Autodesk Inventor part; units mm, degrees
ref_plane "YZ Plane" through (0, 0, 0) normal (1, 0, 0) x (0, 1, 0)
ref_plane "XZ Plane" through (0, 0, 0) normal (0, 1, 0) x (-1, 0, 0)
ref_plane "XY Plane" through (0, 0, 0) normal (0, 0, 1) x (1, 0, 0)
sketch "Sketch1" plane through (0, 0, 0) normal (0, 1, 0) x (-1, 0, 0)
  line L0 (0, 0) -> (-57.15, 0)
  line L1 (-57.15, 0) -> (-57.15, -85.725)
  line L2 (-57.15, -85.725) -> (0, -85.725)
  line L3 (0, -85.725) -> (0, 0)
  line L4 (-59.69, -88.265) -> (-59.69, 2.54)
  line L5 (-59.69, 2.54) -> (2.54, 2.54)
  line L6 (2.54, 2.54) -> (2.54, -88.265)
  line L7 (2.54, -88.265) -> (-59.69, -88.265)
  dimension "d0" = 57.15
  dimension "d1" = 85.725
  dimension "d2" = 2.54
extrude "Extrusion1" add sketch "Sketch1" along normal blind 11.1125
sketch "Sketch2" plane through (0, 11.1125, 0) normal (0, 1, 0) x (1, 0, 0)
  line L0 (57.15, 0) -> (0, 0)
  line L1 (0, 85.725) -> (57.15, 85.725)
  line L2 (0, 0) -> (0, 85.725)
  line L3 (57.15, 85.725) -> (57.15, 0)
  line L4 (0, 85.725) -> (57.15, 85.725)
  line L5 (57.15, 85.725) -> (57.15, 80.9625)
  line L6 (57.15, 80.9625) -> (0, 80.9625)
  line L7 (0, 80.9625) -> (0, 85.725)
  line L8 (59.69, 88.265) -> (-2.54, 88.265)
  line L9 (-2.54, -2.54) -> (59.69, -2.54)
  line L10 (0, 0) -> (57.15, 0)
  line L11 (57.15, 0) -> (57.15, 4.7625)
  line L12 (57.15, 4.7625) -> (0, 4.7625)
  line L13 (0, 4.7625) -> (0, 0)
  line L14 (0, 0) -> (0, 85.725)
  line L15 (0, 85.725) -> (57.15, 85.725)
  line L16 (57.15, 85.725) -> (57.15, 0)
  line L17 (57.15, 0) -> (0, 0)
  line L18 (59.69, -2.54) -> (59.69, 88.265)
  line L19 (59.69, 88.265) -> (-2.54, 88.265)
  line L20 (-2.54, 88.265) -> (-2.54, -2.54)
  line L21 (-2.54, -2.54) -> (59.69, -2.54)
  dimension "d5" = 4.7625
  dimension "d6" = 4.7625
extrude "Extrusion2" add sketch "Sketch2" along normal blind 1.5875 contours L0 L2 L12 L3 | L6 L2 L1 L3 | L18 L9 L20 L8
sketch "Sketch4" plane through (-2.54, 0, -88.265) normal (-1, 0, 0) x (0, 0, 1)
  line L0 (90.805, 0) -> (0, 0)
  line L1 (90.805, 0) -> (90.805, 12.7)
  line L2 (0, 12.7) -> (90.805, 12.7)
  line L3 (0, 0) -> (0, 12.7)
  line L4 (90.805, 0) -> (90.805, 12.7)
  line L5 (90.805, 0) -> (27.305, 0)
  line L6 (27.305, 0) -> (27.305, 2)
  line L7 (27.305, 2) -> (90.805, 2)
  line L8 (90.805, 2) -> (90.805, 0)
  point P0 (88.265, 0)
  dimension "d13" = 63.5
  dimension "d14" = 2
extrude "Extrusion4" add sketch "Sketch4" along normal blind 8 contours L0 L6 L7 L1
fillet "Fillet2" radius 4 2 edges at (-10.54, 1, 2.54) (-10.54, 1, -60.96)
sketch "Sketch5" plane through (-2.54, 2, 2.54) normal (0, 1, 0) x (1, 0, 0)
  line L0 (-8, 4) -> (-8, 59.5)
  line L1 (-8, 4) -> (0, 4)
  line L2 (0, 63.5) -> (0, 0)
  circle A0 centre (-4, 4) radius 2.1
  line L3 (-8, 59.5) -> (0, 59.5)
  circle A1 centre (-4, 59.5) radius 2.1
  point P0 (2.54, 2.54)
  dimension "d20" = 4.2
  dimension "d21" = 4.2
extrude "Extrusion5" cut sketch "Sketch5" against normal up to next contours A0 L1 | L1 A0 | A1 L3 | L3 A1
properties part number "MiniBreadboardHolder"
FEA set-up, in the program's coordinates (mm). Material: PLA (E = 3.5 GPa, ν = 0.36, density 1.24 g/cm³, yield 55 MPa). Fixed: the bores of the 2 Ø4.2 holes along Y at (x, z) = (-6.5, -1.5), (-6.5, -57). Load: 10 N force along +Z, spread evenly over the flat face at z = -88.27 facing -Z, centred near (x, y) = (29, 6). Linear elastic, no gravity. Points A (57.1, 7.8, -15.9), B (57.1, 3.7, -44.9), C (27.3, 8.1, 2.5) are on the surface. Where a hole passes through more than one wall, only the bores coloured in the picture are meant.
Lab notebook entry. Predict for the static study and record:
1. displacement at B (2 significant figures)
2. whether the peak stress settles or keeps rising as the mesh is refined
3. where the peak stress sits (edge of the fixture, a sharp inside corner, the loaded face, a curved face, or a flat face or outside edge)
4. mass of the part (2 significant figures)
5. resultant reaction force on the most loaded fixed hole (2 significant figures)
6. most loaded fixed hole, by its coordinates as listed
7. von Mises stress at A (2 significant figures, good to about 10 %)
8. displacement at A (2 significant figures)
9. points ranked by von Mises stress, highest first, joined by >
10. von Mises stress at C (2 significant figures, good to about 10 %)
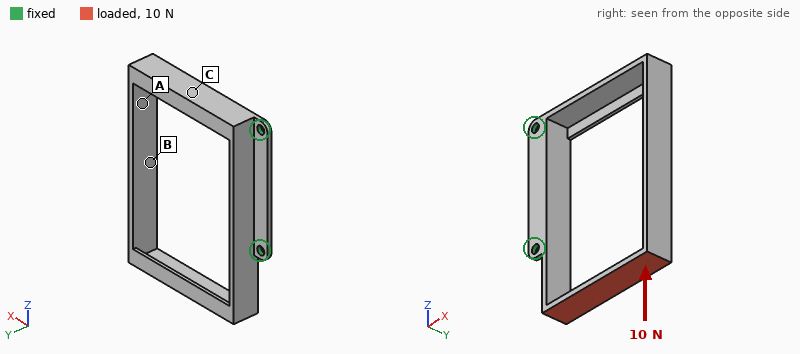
1.2 mm
keeps rising
a sharp inside corner
14 g
7.9 N
(-6.5, -57)
3.0 MPa
1.2 mm
A > C > B
1.6 MPa
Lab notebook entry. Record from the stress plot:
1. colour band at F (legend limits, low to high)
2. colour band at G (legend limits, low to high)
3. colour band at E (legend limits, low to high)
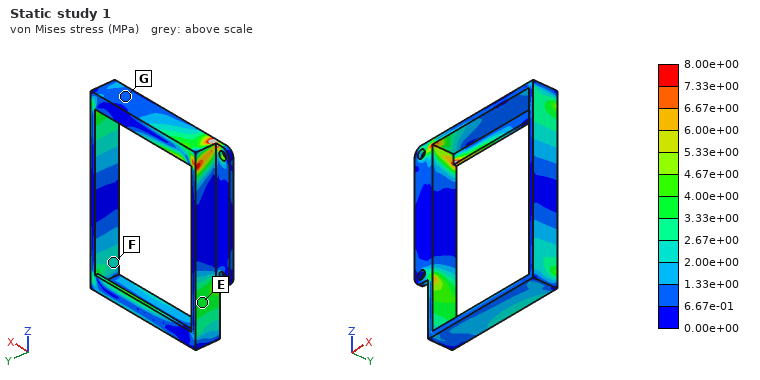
2.00e+00 to 2.67e+00 MPa
6.67e-01 to 1.33e+00 MPa
3.33e+00 to 4.00e+00 MPa
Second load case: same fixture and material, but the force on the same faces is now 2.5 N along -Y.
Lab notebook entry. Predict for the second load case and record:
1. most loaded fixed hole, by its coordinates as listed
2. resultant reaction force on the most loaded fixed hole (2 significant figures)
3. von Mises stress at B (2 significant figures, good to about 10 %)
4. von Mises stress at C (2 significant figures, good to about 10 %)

(-6.5, -57)
4.7 N
0.94 MPa
0.99 MPa
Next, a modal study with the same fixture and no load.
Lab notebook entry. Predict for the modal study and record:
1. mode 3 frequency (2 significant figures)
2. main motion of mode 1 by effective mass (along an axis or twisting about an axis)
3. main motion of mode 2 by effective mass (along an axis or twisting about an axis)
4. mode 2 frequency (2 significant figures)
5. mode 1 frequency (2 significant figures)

220 Hz
along Y
along Z
130 Hz
96 Hz
